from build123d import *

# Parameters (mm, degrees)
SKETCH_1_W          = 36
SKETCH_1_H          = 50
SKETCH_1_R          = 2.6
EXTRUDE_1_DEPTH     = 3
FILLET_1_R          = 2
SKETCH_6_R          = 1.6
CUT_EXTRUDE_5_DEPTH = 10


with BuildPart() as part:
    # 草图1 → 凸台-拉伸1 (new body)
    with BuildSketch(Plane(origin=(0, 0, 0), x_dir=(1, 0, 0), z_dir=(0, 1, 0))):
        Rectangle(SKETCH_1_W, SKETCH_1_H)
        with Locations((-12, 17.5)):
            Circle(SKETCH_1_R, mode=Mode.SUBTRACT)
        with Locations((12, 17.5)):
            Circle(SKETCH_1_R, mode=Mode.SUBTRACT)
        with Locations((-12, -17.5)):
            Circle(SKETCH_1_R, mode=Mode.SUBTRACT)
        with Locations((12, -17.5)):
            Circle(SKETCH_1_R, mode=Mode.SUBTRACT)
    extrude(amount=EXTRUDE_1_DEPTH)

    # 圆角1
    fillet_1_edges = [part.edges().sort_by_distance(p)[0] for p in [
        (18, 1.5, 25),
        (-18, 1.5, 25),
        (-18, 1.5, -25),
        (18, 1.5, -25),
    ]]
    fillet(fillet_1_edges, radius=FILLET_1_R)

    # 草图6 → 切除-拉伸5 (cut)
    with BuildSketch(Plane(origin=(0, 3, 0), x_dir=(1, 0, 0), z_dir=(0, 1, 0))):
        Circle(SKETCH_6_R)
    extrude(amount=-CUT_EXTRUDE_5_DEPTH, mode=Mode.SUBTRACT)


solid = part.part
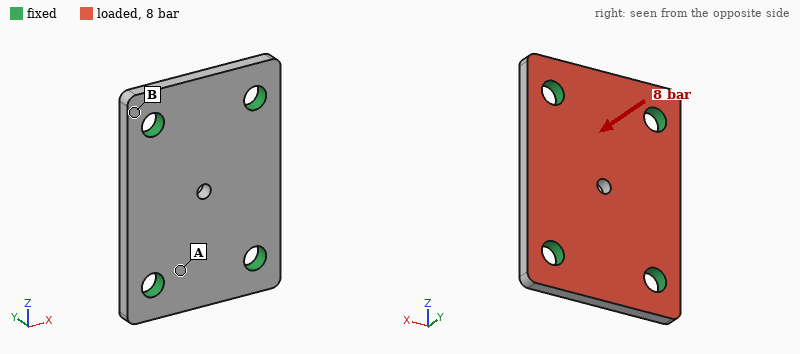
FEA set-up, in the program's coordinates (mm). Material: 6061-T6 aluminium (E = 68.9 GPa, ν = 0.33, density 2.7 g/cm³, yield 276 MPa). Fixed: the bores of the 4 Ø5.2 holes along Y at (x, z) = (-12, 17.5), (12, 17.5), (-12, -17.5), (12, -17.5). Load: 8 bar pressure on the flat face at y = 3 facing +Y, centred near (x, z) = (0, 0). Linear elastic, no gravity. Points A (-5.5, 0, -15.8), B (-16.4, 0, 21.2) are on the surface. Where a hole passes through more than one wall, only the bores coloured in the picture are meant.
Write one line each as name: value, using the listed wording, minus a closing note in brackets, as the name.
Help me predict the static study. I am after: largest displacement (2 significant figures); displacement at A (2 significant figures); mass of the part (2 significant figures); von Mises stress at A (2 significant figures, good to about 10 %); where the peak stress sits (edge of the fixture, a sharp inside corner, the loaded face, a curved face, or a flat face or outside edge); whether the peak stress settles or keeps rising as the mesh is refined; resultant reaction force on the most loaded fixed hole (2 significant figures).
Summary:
largest displacement: 20 µm
displacement at A: 3.6 µm
mass of the part: 14 g
von Mises stress at A: 17 MPa
where the peak stress sits: edge of the fixture
whether the peak stress settles or keeps rising as the mesh is refined: keeps rising
resultant reaction force on the most loaded fixed hole: 340 N
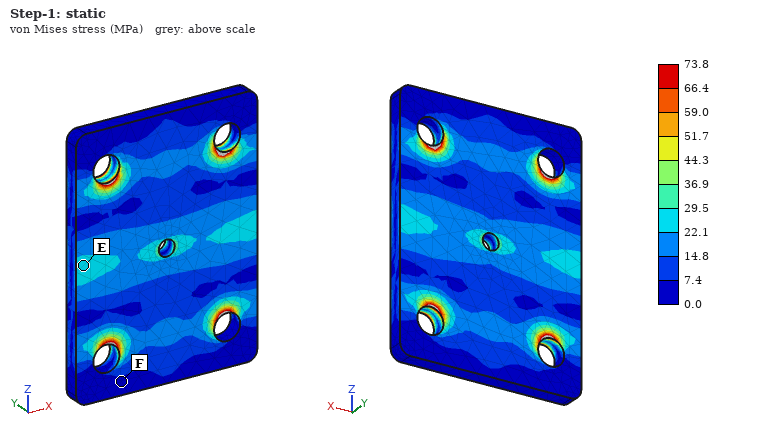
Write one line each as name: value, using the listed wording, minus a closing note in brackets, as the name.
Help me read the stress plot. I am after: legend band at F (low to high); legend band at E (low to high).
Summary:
legend band at F: 0.0 to 7.4 MPa
legend band at E: 22.1 to 29.5 MPa
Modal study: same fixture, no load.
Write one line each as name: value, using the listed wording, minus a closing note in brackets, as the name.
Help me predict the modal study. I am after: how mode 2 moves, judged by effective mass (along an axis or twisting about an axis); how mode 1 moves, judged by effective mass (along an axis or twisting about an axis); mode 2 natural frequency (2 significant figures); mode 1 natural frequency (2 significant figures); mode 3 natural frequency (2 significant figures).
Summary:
how mode 2 moves, judged by effective mass: twisting about Z
how mode 1 moves, judged by effective mass: along Y
mode 2 natural frequency: 17 kHz
mode 1 natural frequency: 13 kHz
mode 3 natural frequency: 22 kHz
